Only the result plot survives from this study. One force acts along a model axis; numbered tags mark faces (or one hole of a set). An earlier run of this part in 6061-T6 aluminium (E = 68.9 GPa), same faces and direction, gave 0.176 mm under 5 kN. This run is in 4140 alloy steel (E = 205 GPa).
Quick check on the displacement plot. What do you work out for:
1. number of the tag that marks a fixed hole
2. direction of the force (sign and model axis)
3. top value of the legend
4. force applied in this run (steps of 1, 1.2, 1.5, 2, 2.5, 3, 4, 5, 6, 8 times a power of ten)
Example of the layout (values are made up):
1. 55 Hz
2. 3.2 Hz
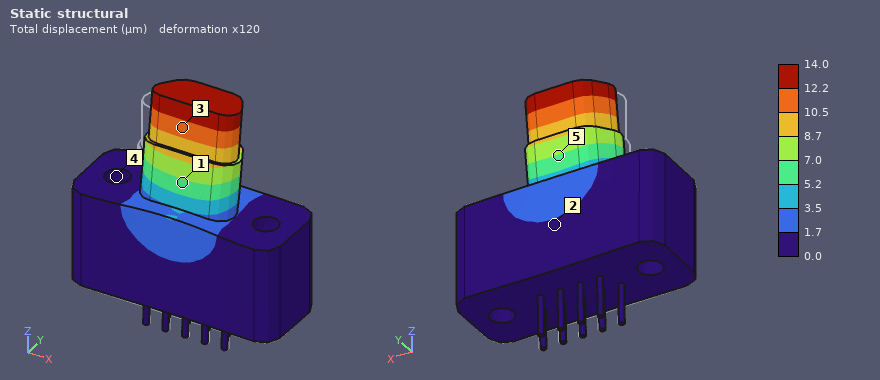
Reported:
1. 4
2. +Y
3. 14.0 µm
4. 1.2 kN
